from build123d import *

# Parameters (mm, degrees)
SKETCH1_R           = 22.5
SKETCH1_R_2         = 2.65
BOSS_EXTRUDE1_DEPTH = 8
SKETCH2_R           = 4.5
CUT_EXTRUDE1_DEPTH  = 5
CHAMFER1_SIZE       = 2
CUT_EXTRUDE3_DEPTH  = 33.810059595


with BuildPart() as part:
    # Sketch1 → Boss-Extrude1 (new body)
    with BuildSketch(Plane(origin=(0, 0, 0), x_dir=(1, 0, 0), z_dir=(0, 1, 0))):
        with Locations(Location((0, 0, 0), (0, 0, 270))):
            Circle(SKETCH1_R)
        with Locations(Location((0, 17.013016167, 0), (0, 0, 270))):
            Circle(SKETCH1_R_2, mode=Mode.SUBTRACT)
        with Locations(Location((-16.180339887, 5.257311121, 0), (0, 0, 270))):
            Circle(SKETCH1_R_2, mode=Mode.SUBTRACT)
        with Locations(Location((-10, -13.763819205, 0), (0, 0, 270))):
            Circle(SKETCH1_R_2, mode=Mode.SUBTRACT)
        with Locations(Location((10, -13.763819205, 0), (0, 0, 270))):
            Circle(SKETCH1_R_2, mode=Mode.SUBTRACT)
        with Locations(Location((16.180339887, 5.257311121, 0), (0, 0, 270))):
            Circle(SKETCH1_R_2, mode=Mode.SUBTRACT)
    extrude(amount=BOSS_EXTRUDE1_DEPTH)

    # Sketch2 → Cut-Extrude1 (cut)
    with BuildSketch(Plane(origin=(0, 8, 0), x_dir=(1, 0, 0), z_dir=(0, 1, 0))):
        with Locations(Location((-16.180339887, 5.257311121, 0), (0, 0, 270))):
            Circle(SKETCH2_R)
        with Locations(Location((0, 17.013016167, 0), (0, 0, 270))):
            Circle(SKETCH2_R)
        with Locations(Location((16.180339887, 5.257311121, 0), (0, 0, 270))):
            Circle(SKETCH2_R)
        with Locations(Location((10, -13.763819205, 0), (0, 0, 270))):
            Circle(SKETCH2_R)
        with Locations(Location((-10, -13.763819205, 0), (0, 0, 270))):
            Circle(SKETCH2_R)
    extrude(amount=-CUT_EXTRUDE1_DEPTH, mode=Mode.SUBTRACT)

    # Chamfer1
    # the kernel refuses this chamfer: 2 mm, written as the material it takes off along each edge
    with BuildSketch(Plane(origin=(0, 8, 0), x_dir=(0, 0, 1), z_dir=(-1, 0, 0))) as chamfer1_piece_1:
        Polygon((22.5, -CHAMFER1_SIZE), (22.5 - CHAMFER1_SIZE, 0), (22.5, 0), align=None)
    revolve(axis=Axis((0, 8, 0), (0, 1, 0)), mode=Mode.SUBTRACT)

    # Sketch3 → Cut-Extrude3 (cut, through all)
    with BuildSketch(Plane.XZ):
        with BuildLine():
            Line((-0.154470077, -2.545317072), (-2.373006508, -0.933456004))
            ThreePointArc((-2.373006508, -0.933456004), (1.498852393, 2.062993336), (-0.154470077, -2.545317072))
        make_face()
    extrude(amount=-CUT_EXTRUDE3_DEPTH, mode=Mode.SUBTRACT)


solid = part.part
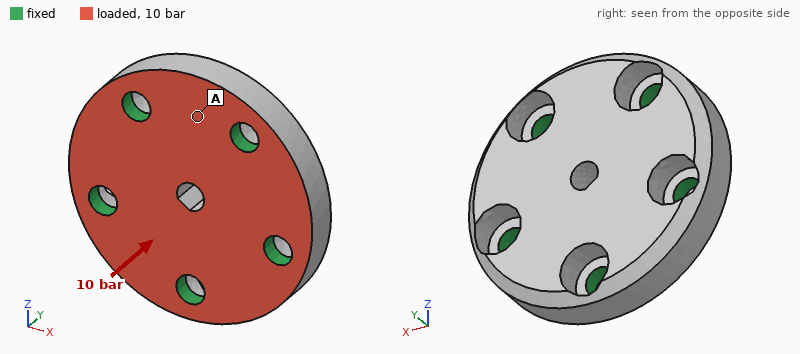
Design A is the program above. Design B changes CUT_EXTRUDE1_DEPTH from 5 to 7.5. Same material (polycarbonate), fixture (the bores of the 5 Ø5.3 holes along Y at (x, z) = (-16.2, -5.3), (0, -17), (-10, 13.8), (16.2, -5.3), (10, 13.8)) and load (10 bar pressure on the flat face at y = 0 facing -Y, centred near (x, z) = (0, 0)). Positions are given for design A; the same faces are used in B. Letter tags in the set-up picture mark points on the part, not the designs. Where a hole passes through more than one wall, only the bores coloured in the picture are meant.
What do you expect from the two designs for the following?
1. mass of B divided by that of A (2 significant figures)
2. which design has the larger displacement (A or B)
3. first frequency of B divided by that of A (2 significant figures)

0.95
B
0.34
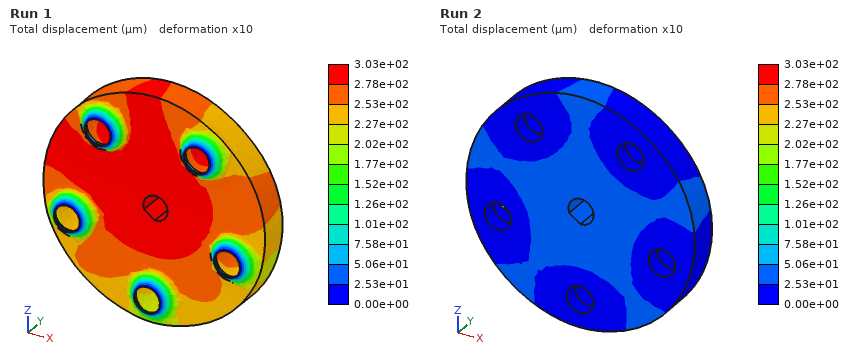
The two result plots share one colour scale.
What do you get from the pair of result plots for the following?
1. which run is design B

Run 1
